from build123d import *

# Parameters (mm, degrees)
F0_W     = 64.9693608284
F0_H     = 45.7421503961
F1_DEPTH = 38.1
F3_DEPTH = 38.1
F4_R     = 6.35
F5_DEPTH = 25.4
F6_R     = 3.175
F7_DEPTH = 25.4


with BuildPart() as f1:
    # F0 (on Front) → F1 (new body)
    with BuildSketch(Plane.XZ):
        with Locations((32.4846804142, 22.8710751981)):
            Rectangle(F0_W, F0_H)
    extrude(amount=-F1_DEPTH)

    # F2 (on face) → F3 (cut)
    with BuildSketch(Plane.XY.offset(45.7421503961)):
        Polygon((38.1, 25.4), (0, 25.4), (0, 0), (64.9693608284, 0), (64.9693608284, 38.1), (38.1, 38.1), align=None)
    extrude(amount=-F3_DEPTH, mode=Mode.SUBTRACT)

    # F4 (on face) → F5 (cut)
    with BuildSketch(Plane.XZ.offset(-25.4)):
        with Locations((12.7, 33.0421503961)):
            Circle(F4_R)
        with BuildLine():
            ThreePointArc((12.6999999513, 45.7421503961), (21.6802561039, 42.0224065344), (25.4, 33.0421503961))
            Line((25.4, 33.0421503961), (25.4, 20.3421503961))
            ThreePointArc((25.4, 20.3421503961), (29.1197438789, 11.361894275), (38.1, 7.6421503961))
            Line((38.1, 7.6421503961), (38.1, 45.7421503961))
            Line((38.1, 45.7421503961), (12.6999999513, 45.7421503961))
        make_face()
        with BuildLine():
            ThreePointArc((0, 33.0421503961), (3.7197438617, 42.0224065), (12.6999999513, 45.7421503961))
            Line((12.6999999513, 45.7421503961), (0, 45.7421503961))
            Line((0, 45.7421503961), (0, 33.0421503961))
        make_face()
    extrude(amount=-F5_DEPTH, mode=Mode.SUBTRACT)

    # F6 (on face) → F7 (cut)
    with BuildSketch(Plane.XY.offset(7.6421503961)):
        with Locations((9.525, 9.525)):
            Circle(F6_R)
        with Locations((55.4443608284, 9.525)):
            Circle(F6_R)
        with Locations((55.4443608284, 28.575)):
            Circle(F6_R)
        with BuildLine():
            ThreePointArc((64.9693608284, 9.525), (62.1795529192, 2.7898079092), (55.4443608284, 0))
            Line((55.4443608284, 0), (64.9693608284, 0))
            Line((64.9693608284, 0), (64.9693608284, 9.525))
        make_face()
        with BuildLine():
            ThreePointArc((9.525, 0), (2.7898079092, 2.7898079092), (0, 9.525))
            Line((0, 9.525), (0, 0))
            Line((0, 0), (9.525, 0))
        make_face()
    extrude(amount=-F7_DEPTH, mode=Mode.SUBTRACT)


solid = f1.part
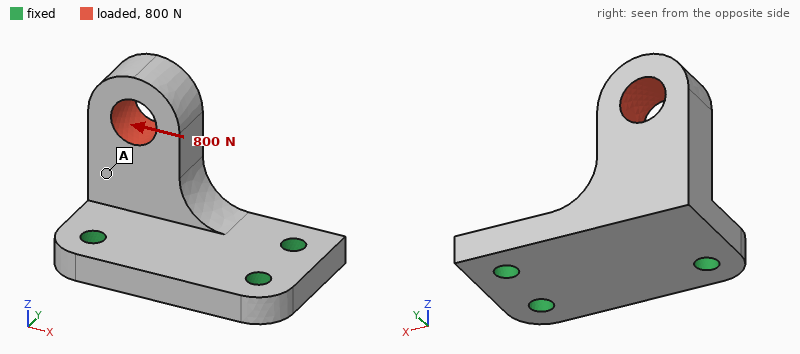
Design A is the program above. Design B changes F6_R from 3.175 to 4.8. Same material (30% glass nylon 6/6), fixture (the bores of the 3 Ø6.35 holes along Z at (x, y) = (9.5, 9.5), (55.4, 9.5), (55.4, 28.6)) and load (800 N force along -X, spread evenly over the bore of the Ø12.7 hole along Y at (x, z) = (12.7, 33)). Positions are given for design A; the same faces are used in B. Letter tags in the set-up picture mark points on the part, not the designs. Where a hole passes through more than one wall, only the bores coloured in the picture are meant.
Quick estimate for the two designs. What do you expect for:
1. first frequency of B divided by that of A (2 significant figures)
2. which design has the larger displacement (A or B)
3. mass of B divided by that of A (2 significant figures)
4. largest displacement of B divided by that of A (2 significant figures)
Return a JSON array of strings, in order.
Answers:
["1.1", "A", "0.97", "0.87"]
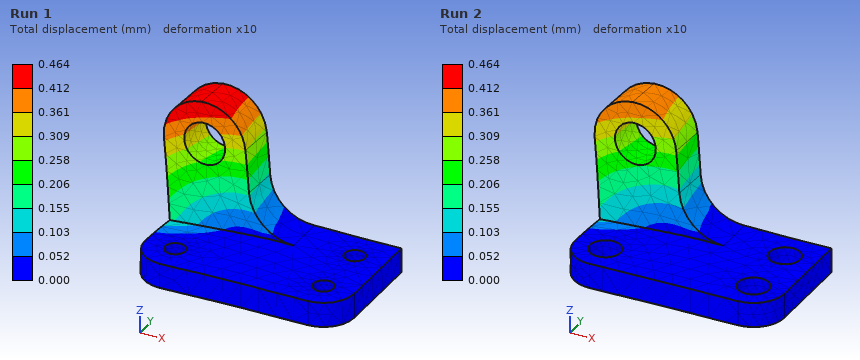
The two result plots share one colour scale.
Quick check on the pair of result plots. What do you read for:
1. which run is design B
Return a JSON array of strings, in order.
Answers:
["Run 2"]
